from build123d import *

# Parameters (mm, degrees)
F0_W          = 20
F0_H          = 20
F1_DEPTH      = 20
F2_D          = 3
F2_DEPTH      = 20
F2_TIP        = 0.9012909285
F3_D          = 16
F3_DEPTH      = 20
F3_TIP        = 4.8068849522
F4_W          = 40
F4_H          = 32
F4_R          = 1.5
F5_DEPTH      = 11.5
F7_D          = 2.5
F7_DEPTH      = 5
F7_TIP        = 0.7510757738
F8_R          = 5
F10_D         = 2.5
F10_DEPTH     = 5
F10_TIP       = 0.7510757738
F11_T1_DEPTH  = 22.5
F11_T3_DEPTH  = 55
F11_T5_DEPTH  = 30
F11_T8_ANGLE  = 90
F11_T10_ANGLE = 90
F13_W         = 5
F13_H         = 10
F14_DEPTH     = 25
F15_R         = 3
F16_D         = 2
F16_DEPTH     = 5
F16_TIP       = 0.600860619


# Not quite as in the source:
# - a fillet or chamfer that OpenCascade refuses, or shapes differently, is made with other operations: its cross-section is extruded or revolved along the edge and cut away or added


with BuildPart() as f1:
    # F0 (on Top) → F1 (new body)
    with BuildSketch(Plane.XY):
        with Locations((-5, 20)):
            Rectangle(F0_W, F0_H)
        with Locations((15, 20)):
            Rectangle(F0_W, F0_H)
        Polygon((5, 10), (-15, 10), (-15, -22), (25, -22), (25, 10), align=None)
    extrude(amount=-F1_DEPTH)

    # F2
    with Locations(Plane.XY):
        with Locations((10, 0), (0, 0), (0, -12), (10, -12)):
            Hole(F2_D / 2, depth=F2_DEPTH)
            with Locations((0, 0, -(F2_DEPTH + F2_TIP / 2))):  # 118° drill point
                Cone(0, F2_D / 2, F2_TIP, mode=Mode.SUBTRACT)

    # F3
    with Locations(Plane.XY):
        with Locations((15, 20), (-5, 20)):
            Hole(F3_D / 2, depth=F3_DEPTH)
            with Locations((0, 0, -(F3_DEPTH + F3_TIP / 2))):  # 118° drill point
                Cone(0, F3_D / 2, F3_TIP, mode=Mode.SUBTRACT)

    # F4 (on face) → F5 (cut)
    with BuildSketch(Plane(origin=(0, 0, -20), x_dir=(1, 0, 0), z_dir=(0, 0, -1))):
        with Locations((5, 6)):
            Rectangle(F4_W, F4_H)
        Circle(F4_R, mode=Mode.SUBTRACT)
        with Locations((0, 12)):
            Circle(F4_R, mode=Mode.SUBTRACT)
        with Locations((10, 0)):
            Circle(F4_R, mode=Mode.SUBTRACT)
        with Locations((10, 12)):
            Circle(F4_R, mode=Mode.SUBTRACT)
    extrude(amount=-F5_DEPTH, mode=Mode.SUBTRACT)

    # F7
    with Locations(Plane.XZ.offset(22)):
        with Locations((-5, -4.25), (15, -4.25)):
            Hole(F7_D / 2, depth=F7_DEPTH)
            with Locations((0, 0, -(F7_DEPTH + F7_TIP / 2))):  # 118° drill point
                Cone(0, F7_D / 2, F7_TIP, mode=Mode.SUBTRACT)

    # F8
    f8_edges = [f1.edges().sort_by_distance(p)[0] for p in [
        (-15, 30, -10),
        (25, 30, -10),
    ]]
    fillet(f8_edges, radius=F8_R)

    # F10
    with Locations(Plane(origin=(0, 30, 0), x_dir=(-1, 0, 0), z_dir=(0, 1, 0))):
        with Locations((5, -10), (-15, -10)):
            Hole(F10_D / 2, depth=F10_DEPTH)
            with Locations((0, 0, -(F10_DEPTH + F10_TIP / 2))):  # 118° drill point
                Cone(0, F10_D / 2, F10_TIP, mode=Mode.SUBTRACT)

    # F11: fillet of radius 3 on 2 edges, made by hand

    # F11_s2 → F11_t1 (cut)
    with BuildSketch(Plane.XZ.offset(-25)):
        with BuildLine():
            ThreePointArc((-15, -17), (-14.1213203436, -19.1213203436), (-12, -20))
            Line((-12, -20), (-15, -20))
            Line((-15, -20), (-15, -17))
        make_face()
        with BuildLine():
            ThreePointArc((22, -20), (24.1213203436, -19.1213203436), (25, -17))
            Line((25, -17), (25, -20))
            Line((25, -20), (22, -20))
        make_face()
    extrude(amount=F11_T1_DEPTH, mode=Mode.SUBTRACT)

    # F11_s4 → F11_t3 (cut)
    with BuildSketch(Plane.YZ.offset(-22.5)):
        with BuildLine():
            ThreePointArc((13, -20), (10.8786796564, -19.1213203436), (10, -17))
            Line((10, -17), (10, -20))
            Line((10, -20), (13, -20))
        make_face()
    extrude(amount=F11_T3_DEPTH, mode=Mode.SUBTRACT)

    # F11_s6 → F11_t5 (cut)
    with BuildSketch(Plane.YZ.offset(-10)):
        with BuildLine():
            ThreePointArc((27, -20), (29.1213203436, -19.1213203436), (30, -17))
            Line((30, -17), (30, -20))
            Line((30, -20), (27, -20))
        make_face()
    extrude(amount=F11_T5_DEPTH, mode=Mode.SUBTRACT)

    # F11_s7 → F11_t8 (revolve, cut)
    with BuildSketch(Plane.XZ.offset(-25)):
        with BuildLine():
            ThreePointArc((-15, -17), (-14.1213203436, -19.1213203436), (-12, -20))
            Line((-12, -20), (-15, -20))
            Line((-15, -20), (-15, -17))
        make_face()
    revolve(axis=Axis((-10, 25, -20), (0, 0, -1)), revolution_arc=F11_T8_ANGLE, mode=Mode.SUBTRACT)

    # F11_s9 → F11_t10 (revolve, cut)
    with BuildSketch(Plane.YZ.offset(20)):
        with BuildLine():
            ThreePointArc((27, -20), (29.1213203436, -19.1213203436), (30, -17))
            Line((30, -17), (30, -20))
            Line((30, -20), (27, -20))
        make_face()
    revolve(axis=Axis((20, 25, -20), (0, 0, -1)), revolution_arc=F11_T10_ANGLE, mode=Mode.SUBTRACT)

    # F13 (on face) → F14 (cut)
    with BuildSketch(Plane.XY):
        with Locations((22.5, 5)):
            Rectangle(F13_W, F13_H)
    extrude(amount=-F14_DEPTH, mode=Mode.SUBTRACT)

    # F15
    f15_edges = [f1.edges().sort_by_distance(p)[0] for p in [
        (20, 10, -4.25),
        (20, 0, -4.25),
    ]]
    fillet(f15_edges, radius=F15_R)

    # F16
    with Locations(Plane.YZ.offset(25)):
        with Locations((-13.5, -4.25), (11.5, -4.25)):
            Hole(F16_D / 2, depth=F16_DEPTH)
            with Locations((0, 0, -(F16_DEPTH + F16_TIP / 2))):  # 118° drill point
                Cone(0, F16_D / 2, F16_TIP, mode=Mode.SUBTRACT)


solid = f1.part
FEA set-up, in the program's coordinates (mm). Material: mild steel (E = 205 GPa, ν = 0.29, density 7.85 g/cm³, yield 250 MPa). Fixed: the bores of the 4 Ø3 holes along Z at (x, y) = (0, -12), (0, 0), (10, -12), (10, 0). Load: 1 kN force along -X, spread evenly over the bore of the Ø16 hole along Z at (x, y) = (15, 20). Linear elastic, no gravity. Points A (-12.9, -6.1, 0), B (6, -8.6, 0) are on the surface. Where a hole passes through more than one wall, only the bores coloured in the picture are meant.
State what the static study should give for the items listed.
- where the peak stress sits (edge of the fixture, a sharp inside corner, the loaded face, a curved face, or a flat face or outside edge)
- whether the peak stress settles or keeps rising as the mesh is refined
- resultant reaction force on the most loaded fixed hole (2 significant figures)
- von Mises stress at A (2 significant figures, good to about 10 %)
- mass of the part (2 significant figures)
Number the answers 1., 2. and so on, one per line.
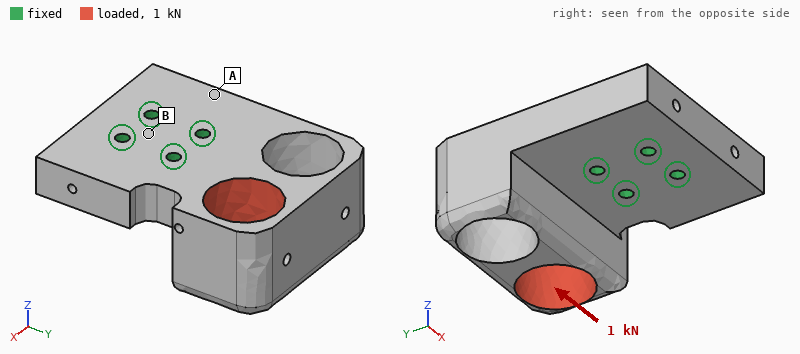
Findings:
1. edge of the fixture
2. keeps rising
3. 1.1 kN
4. 7.5 MPa
5. 140 g
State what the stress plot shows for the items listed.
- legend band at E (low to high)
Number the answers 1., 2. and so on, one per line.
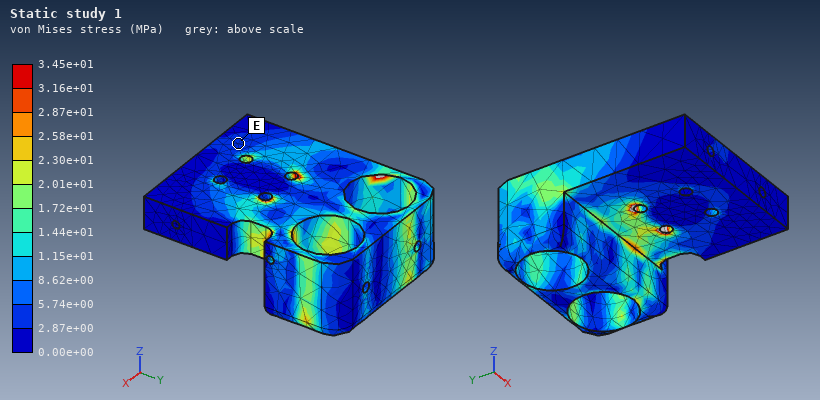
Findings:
1. 2.87e+00 to 5.74e+00 MPa
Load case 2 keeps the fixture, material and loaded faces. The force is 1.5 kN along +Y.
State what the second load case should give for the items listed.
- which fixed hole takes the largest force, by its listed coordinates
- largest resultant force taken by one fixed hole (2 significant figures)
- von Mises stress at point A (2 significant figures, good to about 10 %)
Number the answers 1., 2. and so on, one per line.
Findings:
1. (10, 0)
2. 1.2 kN
3. 6.3 MPa
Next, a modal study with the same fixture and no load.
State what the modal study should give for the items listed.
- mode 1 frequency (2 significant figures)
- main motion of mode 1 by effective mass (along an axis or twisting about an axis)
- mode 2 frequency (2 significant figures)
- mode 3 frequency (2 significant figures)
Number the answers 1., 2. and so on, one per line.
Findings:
1. 5200 Hz
2. along Z
3. 8200 Hz
4. 8500 Hz
